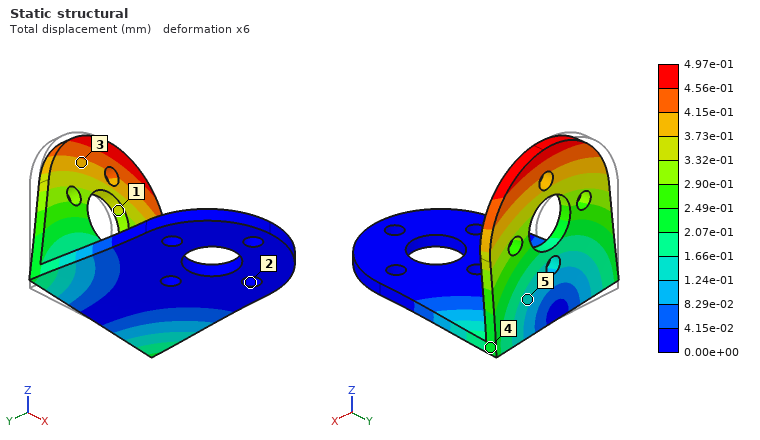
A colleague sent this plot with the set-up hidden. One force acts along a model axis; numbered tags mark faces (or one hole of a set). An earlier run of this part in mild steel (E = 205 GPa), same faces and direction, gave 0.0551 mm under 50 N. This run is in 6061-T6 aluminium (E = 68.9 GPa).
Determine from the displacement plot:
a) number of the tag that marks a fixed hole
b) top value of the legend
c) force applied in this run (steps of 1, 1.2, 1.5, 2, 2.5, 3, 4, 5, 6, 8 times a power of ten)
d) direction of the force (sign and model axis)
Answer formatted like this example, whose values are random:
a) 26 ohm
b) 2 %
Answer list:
a) 2
b) 4.97e-01 mm
c) 150 N
d) +X
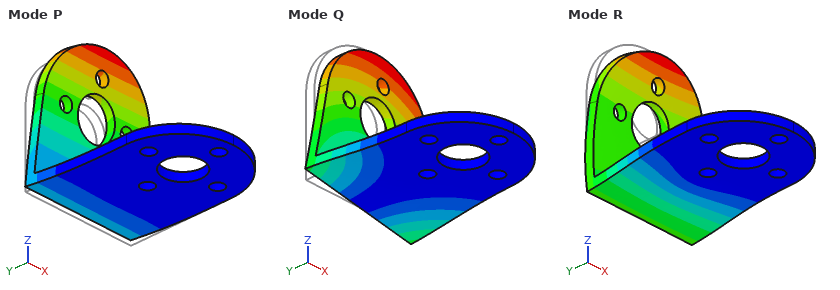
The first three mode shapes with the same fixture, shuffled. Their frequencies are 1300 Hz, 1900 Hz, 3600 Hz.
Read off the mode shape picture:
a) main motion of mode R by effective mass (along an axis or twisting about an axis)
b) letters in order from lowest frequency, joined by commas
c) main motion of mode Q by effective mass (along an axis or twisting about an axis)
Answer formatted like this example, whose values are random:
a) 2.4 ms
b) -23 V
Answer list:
a) along Z
b) P, Q, R
c) along X
